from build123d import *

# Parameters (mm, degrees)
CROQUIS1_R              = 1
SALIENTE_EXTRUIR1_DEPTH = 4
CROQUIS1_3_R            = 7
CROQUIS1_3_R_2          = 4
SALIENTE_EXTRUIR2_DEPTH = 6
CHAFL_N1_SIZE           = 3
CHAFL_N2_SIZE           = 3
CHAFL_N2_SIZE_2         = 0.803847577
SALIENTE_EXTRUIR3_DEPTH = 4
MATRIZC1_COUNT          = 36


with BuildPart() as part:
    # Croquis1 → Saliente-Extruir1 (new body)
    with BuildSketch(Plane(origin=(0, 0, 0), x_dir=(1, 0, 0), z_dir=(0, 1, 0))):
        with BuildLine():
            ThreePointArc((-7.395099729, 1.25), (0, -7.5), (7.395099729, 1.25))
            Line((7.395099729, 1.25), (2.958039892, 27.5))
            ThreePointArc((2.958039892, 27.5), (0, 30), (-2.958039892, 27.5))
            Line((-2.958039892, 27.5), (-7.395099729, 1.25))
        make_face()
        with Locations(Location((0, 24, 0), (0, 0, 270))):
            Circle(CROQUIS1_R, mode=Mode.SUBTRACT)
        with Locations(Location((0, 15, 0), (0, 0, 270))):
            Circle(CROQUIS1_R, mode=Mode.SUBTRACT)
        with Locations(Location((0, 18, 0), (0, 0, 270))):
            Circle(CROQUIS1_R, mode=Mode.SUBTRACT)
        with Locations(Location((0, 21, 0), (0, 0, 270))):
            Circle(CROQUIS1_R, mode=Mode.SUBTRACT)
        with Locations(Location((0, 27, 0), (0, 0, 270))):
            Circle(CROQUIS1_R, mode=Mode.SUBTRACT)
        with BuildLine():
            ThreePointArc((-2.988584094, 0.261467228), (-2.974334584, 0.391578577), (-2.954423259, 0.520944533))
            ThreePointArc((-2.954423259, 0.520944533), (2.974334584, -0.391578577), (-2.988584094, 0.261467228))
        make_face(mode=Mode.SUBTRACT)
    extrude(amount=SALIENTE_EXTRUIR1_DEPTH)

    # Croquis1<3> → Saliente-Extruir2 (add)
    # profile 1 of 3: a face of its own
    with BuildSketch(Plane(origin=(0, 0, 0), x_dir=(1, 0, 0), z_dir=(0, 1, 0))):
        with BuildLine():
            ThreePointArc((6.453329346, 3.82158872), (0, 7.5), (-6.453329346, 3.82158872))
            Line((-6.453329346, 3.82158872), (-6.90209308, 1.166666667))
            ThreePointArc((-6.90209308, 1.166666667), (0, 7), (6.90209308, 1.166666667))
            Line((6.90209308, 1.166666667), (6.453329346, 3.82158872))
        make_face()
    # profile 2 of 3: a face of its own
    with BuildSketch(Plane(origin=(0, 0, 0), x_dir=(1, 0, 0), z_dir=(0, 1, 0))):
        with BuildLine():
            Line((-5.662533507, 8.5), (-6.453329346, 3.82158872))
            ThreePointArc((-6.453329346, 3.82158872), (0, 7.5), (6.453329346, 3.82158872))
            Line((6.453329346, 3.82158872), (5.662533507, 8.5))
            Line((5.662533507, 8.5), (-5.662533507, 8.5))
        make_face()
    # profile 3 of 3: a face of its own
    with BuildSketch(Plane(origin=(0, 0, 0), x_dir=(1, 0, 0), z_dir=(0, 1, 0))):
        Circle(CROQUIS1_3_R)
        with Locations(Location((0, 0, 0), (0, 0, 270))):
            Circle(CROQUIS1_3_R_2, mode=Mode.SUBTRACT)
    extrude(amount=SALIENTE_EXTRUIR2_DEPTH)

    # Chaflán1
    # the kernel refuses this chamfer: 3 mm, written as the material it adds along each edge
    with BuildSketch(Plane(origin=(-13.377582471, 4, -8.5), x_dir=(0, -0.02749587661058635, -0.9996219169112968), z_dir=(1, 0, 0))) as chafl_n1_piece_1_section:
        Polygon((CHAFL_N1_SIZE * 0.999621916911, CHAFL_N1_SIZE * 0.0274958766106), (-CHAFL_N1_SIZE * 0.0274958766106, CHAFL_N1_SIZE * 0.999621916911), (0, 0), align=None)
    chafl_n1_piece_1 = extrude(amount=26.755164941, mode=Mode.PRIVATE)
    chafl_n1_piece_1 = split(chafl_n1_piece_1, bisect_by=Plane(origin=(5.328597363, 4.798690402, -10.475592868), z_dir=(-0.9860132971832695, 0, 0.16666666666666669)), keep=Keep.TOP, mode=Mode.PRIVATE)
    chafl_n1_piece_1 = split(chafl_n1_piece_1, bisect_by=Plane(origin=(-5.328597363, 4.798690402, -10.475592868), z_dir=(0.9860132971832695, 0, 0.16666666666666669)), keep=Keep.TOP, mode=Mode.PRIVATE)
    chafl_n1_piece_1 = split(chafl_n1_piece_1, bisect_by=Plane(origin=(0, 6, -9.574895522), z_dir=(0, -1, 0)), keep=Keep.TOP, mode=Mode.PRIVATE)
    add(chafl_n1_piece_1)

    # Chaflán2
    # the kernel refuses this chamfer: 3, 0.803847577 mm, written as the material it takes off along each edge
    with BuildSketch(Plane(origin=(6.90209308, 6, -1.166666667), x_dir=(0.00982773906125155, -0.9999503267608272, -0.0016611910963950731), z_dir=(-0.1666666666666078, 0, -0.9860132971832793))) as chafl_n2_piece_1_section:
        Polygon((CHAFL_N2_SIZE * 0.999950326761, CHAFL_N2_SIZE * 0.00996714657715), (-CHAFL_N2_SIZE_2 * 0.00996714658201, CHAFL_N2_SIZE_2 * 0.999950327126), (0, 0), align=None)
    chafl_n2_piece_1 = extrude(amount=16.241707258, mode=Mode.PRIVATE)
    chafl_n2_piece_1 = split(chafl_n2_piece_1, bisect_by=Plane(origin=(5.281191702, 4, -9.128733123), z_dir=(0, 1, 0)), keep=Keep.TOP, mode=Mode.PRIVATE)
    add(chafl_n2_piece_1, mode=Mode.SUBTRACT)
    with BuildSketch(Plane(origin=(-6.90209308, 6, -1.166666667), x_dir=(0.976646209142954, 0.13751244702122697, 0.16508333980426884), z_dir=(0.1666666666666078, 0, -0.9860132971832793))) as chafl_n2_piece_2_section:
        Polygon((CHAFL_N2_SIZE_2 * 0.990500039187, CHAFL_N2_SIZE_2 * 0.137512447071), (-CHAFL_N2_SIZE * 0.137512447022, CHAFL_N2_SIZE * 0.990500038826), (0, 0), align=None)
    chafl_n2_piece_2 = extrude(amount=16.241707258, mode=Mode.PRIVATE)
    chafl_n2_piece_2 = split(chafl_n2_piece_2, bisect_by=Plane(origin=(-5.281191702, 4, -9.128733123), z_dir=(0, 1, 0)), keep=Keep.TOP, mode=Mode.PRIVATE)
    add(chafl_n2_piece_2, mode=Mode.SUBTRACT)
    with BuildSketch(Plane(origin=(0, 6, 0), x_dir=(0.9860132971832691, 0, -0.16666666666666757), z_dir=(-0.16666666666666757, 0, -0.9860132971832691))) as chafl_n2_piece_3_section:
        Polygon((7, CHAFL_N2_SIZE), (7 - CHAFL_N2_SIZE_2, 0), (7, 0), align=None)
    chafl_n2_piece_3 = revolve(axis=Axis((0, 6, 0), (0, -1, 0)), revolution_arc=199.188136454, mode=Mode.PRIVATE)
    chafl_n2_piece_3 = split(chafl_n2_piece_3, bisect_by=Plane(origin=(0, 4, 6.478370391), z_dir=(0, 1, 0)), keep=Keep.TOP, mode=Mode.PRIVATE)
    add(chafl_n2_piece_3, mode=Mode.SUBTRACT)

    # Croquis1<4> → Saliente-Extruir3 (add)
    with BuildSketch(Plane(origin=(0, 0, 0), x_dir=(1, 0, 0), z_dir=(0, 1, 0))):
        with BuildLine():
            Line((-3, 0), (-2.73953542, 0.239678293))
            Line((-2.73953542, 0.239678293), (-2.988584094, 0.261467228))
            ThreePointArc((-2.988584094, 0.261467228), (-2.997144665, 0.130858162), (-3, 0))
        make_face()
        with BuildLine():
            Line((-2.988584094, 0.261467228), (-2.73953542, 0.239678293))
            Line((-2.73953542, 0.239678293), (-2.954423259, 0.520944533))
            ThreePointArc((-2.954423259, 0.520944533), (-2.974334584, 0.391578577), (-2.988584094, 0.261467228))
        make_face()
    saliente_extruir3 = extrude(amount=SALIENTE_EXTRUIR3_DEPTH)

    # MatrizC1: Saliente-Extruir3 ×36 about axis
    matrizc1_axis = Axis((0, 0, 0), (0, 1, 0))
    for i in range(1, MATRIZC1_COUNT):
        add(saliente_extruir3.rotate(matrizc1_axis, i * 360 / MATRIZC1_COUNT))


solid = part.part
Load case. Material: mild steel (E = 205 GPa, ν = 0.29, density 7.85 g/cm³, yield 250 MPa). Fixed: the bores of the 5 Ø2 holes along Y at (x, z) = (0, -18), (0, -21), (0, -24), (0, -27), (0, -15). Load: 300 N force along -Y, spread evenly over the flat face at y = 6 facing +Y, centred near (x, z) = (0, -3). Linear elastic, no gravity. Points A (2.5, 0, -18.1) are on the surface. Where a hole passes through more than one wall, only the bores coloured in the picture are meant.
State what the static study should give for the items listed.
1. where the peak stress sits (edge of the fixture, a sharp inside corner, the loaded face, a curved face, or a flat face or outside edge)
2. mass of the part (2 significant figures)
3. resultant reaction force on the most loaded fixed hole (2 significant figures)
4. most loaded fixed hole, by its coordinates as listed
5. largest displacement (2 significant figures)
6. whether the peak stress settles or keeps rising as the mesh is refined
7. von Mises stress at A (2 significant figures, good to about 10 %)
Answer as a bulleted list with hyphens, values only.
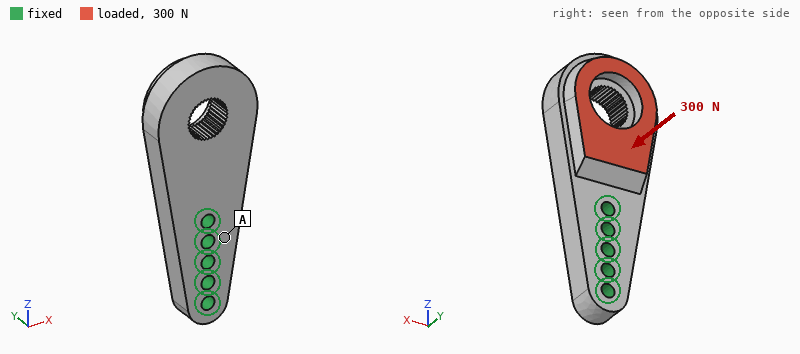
- edge of the fixture
- 13 g
- 530 N
- (0, -15)
- 34 µm
- keeps rising
- 21 MPa
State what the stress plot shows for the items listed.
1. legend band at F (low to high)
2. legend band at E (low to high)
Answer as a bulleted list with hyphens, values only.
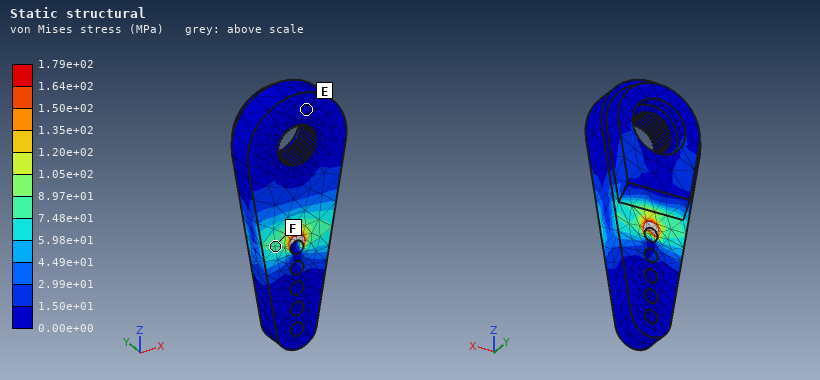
- 7.48e+01 to 8.97e+01 MPa
- 0.00e+00 to 1.50e+01 MPa
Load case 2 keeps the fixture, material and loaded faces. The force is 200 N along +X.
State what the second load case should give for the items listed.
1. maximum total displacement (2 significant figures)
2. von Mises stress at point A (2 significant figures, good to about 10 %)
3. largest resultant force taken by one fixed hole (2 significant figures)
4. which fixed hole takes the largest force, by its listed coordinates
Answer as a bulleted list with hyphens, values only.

- 8.2 µm
- 23 MPa
- 480 N
- (0, -15)
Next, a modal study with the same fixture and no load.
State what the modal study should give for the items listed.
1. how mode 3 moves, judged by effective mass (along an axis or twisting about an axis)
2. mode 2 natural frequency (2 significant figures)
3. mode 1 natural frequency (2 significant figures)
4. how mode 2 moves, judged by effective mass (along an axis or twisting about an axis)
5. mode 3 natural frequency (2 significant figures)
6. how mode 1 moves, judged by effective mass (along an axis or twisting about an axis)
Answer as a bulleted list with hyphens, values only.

- twisting about Z
- 10 kHz
- 6300 Hz
- along X
- 18 kHz
- along Y
